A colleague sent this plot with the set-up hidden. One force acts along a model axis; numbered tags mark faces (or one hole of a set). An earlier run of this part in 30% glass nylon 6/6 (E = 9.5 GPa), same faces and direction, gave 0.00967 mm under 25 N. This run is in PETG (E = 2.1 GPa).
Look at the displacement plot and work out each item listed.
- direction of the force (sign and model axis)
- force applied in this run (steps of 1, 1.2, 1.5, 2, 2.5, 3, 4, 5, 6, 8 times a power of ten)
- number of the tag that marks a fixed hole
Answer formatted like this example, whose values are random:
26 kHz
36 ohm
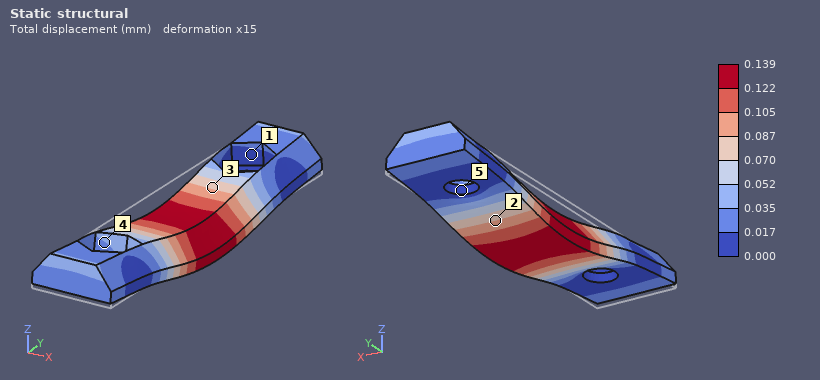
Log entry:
-Z
80 N
5
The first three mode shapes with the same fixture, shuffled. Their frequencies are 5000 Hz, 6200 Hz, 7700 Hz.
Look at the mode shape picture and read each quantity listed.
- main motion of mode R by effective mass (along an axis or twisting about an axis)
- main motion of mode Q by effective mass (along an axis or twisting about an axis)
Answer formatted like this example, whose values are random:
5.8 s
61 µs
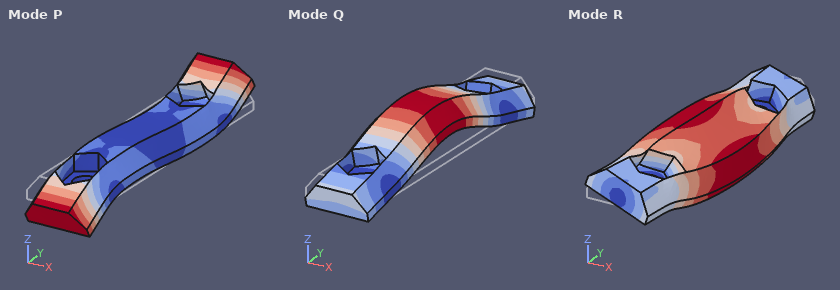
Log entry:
along X
along Z
